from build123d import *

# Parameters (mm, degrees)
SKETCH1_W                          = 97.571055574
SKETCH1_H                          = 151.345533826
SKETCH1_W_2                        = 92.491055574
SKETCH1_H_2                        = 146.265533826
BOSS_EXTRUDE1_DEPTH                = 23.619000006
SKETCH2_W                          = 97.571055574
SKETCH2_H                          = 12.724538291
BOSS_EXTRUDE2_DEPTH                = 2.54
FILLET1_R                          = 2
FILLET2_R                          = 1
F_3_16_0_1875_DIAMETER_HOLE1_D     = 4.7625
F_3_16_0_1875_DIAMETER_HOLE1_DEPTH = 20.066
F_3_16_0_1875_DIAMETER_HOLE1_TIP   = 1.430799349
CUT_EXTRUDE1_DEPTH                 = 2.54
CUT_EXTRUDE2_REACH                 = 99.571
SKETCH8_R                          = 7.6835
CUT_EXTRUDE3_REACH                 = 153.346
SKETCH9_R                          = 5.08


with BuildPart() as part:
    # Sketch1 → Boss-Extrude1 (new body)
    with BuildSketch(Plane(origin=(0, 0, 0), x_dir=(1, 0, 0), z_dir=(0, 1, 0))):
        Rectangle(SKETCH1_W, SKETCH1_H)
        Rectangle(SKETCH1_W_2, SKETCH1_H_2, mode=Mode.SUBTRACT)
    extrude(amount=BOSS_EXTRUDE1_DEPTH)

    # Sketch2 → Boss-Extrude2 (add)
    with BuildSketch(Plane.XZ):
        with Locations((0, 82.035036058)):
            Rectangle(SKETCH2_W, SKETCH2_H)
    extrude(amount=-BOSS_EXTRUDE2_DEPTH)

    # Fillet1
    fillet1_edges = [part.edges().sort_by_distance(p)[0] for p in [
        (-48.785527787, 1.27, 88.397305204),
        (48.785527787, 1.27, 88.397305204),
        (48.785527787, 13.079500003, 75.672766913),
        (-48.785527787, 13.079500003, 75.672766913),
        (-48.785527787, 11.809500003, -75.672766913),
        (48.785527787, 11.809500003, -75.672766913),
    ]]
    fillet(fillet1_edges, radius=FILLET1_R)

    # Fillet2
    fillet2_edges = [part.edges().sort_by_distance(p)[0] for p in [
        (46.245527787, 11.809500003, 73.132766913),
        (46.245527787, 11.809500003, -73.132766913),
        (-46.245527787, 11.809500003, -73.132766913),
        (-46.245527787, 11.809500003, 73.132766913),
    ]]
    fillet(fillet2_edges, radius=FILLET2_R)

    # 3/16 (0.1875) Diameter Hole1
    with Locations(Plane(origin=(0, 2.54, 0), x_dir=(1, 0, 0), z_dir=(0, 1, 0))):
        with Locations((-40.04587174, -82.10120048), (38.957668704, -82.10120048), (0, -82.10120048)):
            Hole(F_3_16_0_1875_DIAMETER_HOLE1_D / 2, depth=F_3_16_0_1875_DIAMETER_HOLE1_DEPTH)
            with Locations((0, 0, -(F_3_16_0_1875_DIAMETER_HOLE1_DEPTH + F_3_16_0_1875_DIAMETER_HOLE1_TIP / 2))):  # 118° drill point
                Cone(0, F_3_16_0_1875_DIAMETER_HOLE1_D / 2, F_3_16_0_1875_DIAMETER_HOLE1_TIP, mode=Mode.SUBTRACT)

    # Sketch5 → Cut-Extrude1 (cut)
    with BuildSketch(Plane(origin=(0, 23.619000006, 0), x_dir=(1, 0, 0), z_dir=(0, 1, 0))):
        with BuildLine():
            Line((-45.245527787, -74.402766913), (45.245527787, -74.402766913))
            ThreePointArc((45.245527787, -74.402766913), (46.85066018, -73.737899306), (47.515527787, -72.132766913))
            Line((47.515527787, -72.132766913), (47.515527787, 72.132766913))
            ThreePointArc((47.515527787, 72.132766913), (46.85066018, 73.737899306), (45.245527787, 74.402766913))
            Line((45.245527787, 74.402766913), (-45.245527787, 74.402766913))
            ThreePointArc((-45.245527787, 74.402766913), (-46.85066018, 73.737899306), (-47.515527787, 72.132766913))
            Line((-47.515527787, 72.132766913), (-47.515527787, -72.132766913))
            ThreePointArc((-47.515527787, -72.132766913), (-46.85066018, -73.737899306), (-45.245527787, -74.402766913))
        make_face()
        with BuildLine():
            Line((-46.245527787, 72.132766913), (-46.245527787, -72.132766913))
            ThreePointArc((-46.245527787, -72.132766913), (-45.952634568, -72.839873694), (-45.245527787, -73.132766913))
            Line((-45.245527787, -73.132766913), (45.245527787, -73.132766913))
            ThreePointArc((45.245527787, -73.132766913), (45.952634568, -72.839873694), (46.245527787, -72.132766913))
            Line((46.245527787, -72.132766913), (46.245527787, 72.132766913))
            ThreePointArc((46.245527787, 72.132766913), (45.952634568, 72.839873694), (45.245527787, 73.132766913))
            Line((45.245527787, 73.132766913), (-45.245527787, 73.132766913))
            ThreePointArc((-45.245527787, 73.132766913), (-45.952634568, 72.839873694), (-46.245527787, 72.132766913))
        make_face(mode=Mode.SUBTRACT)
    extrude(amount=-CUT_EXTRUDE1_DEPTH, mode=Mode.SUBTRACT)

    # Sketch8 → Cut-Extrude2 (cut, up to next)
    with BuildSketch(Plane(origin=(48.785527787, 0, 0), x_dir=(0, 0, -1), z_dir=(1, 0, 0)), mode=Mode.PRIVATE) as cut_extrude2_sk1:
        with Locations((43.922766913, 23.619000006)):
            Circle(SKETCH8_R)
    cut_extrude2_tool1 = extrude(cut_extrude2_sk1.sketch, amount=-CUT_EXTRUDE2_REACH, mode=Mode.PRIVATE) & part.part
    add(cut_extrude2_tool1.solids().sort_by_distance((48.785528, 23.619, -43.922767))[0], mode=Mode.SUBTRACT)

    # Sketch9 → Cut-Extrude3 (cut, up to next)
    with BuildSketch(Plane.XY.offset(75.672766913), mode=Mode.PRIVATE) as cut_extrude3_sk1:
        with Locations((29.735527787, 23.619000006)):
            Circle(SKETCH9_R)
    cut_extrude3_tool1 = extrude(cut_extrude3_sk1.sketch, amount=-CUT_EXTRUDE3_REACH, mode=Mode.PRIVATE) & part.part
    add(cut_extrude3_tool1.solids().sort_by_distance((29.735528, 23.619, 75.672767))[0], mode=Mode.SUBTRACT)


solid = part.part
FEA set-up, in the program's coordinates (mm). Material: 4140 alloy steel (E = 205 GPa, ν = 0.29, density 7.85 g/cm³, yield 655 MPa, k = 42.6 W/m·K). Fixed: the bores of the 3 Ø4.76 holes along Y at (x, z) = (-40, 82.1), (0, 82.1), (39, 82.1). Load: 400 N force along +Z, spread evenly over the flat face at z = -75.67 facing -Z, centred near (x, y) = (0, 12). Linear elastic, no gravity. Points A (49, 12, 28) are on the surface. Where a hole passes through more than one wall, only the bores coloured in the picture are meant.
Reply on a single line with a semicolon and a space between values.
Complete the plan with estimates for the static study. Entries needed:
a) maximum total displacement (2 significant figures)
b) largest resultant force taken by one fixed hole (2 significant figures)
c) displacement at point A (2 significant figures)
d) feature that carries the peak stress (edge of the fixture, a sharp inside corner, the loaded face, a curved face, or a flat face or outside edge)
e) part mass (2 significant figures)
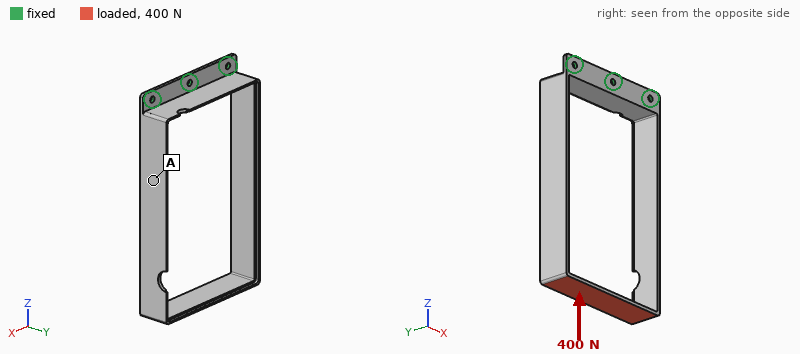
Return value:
0.72 mm; 270 N; 0.23 mm; a flat face or outside edge; 240 g
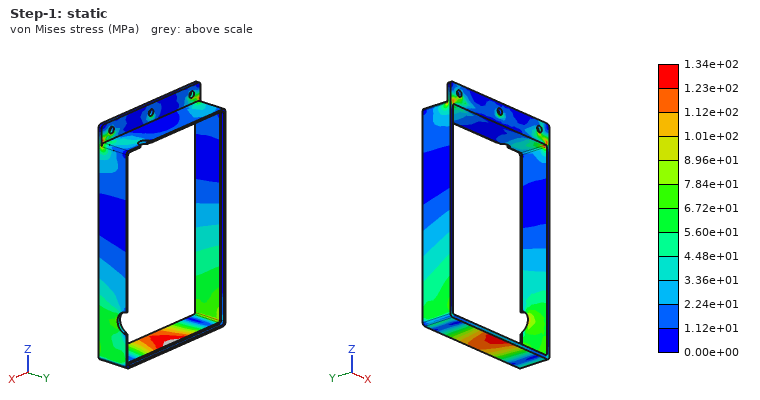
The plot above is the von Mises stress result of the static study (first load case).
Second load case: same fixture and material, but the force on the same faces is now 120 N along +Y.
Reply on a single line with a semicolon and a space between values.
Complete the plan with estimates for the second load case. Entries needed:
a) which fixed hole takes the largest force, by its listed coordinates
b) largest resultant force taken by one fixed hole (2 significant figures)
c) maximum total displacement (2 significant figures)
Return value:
(0, 82.1); 560 N; 2.2 mm
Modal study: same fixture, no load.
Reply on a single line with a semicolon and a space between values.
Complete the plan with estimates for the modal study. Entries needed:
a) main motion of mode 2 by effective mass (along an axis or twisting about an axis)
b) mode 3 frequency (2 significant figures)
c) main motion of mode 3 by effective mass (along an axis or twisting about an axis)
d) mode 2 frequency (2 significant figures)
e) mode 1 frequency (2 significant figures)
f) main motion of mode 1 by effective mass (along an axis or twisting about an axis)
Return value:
along Y; 240 Hz; twisting about Z; 130 Hz; 98 Hz; along X
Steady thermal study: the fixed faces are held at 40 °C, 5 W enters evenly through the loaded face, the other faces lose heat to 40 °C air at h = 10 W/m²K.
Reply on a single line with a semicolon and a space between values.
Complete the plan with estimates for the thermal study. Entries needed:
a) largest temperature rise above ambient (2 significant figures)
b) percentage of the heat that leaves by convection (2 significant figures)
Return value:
64 K; 88 %
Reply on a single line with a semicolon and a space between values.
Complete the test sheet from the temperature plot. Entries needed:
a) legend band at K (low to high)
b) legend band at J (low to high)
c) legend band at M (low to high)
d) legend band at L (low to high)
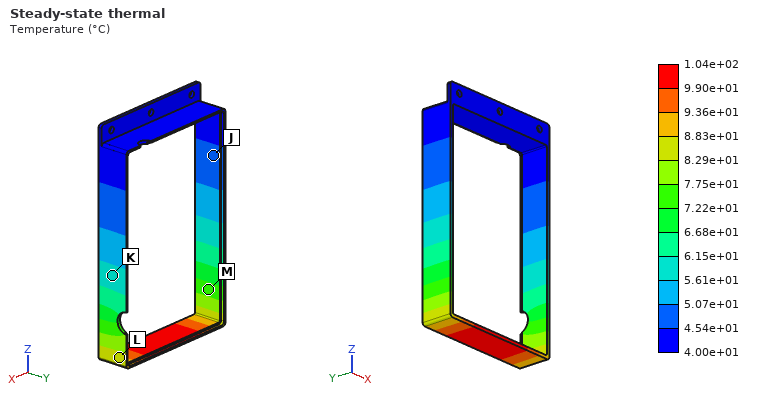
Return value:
5.61e+01 to 6.15e+01 °C; 4.54e+01 to 5.07e+01 °C; 7.22e+01 to 7.75e+01 °C; 8.29e+01 to 8.83e+01 °C
